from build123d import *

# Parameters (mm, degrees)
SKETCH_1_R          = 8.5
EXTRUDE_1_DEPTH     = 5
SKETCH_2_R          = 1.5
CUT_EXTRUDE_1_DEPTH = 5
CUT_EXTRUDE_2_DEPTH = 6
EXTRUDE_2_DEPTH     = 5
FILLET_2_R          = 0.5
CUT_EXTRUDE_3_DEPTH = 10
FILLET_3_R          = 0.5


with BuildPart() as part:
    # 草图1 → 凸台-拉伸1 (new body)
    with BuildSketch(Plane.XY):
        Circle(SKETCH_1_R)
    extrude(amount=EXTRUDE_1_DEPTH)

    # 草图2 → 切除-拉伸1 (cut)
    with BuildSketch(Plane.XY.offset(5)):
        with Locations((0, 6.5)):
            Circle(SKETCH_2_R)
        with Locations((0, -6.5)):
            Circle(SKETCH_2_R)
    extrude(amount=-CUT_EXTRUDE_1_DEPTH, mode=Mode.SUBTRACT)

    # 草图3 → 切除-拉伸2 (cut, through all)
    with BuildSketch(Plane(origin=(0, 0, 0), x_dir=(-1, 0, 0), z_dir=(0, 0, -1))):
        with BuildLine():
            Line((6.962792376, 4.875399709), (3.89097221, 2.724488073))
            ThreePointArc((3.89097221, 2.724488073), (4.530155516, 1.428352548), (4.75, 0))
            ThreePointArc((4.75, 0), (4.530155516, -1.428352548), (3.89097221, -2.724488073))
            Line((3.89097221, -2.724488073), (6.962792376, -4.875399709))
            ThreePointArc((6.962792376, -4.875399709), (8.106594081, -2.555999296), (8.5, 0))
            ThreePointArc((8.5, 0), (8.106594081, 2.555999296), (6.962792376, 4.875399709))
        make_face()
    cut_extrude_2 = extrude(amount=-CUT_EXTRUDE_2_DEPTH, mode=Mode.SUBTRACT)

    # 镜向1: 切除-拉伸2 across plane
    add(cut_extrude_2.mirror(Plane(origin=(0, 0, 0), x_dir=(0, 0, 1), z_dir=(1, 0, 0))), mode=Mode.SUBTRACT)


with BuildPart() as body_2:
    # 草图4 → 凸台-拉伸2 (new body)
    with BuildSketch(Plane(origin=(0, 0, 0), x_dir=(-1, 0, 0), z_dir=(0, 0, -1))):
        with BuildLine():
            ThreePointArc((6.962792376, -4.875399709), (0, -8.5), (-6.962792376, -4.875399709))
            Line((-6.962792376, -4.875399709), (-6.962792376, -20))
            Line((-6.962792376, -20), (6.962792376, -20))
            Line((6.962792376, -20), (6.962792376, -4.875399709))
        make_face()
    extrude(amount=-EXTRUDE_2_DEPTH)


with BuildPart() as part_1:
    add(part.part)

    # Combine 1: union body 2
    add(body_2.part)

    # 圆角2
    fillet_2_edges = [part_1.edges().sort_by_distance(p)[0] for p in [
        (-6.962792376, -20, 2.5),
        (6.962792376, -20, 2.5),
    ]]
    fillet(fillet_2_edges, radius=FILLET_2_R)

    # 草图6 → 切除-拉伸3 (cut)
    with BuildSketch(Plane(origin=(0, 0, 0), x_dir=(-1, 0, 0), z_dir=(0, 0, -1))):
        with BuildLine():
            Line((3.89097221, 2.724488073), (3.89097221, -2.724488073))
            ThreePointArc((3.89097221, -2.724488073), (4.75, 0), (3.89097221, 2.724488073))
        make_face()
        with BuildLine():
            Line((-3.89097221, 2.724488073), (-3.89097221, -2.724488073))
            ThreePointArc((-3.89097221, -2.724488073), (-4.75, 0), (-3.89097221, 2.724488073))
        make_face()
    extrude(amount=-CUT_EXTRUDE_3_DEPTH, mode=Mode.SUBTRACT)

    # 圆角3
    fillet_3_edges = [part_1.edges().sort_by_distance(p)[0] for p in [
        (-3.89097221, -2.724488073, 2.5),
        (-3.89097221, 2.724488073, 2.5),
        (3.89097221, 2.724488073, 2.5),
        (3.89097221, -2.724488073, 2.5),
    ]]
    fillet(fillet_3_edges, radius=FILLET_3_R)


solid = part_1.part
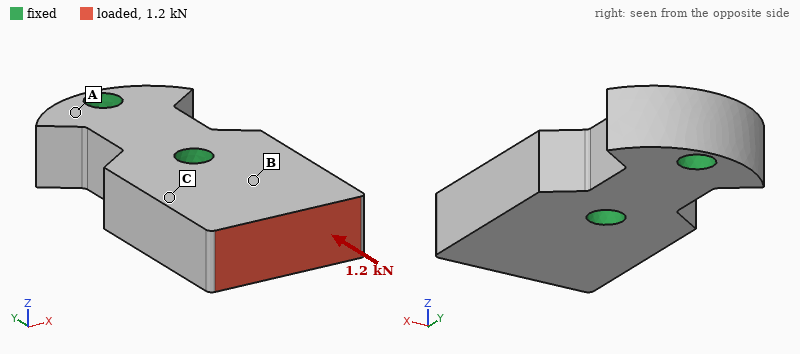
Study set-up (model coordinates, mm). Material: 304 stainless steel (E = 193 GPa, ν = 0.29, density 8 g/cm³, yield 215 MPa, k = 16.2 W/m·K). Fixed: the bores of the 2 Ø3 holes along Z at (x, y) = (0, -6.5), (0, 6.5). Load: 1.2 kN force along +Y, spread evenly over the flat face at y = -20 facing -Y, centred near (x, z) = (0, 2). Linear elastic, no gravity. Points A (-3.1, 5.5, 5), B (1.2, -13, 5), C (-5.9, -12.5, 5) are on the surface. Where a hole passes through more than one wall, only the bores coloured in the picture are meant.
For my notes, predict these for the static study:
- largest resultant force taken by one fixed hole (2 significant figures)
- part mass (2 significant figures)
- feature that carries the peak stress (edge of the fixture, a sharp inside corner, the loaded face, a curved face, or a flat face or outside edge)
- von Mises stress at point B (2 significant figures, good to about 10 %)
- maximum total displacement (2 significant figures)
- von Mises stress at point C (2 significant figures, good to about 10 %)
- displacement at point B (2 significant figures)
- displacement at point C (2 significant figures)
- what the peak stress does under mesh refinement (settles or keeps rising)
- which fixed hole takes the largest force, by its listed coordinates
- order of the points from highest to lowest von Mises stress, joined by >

1.1 kN
13 g
edge of the fixture
23 MPa
1.5 µm
13 MPa
0.78 µm
0.87 µm
keeps rising
(0, -6.5)
B > C > A
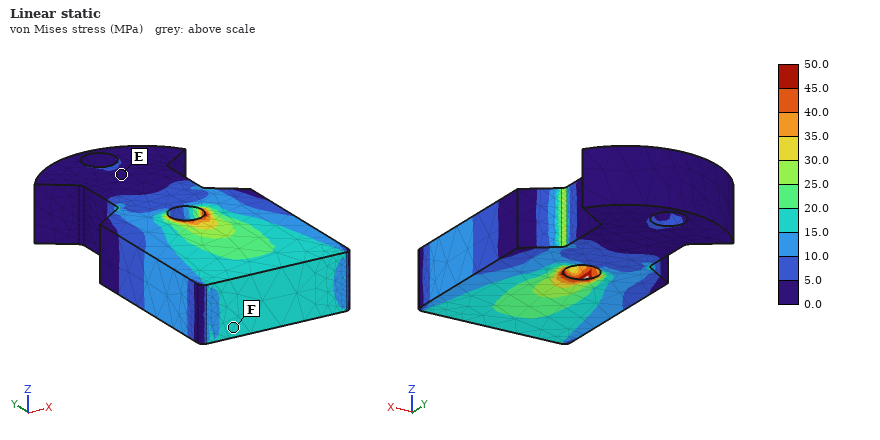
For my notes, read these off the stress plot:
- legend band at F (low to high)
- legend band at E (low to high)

15.0 to 20.0 MPa
0.0 to 5.0 MPa
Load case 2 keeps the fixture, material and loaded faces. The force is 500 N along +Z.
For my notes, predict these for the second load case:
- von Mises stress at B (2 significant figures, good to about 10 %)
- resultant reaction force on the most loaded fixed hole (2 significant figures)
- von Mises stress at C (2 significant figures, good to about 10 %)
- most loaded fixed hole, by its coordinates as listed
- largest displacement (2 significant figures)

59 MPa
590 N
59 MPa
(0, -6.5)
18 µm
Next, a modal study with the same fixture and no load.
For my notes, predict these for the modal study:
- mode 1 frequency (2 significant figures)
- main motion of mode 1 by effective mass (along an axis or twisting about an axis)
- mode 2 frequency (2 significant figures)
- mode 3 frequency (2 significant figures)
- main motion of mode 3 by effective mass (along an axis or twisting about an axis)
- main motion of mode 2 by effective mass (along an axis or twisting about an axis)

19 kHz
along Z
24 kHz
32 kHz
twisting about Y
along X
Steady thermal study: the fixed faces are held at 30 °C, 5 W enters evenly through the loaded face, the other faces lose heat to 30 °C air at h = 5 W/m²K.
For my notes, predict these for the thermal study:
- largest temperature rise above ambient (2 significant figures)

63 K
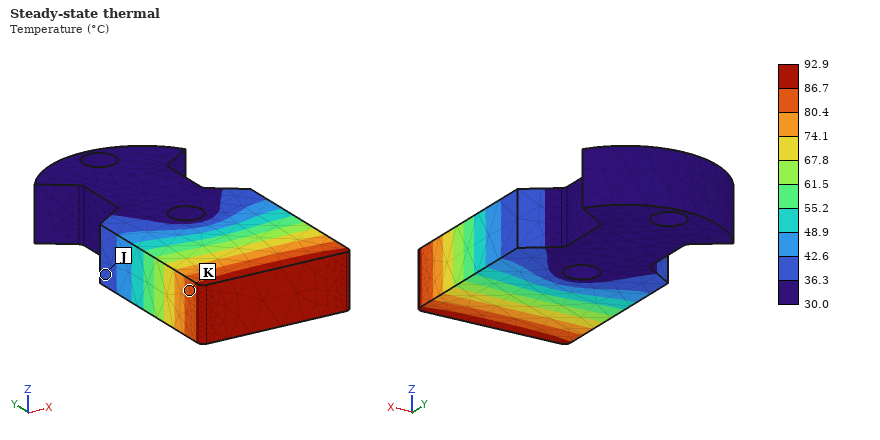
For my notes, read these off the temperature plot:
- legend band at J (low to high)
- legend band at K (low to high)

36.3 to 42.6 °C
80.4 to 86.7 °C
